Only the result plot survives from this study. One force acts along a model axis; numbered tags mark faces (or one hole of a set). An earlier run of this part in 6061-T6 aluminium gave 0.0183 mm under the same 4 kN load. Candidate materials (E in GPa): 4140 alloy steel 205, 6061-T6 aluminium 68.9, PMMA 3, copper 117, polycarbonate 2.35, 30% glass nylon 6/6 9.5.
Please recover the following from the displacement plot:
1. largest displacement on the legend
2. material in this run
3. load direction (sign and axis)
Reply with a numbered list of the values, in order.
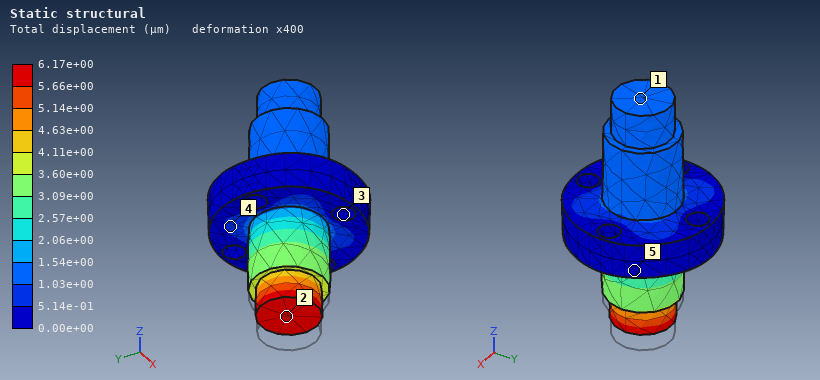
1. 6.17e+00 µm
2. 4140 alloy steel
3. +Z
